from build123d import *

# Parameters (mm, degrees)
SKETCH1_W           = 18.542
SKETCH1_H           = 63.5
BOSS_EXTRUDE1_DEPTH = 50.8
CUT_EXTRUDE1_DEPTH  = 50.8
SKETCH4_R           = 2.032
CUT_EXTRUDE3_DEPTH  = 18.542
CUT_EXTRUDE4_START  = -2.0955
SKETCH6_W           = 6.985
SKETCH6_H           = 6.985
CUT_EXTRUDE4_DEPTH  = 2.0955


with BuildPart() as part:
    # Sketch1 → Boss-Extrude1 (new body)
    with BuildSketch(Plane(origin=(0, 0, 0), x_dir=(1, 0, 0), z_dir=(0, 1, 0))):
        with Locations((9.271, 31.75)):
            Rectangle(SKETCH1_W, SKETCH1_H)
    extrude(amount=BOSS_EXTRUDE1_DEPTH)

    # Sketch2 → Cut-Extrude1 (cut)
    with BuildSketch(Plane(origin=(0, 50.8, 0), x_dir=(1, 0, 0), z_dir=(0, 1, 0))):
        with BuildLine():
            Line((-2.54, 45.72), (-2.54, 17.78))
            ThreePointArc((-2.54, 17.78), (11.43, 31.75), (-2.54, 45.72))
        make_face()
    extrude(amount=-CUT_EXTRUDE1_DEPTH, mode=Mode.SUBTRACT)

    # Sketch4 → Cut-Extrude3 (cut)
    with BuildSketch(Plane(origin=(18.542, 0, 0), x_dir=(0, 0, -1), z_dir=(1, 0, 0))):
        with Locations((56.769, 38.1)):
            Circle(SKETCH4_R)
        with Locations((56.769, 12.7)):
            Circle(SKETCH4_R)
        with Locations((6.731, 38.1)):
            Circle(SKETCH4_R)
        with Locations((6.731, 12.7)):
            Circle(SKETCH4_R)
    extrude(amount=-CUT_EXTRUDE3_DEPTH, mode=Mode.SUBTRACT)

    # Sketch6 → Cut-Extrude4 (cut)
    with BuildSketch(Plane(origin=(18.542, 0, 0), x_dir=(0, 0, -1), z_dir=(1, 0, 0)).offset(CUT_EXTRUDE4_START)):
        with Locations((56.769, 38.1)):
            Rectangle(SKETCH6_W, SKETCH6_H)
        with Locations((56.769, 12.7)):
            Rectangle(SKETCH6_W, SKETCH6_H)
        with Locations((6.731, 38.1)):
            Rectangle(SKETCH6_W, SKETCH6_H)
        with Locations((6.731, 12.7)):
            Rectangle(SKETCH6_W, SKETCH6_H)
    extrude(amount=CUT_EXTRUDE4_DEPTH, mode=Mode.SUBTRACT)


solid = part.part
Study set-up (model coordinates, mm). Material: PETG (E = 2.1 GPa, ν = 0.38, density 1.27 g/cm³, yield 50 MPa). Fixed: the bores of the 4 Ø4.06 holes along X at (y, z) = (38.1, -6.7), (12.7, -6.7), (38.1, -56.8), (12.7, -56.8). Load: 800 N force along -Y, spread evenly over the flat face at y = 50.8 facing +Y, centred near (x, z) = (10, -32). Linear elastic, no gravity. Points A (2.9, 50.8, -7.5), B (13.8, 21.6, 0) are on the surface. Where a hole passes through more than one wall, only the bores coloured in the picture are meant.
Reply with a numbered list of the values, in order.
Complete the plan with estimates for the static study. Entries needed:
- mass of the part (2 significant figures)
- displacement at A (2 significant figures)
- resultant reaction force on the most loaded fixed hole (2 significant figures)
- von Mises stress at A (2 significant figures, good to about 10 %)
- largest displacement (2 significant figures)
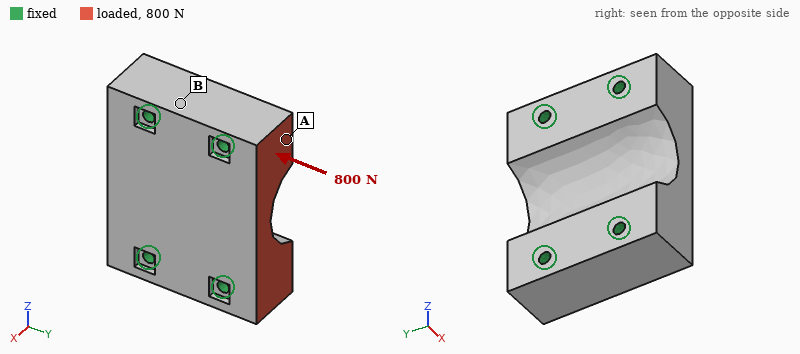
1. 59 g
2. 7.5 µm
3. 300 N
4. 1.0 MPa
5. 20 µm
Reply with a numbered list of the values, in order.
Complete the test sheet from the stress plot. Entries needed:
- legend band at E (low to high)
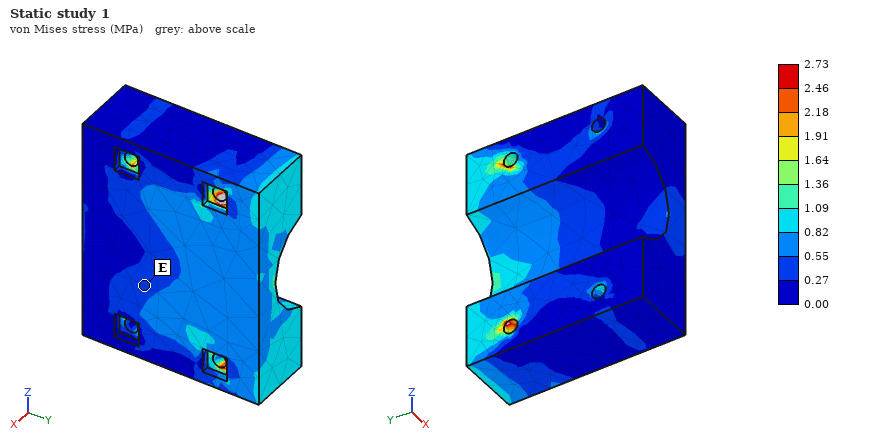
1. 0.27 to 0.55 MPa
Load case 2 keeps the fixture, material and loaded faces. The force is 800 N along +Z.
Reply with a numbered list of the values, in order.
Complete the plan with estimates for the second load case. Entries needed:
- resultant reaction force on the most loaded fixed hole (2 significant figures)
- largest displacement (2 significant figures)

1. 430 N
2. 38 µm
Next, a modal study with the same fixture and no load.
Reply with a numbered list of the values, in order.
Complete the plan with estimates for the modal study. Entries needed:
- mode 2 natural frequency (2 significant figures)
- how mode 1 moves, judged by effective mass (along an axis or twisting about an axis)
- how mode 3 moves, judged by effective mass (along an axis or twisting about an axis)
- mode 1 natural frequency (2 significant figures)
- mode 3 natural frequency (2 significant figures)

1. 5700 Hz
2. along X
3. along Y
4. 5400 Hz
5. 7500 Hz
